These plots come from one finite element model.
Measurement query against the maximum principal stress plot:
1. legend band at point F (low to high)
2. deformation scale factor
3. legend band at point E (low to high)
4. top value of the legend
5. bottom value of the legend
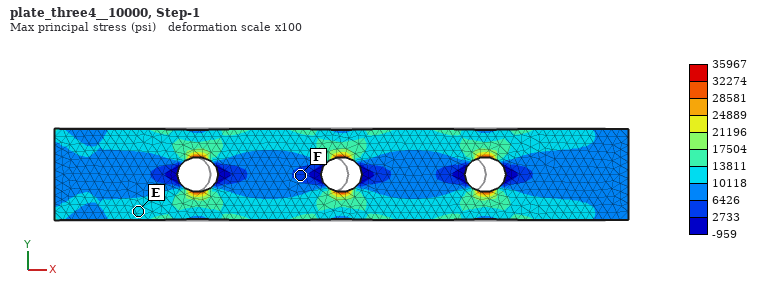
2733 to 6426 psi
100
10118 to 13811 psi
35967 psi
-959 psi
